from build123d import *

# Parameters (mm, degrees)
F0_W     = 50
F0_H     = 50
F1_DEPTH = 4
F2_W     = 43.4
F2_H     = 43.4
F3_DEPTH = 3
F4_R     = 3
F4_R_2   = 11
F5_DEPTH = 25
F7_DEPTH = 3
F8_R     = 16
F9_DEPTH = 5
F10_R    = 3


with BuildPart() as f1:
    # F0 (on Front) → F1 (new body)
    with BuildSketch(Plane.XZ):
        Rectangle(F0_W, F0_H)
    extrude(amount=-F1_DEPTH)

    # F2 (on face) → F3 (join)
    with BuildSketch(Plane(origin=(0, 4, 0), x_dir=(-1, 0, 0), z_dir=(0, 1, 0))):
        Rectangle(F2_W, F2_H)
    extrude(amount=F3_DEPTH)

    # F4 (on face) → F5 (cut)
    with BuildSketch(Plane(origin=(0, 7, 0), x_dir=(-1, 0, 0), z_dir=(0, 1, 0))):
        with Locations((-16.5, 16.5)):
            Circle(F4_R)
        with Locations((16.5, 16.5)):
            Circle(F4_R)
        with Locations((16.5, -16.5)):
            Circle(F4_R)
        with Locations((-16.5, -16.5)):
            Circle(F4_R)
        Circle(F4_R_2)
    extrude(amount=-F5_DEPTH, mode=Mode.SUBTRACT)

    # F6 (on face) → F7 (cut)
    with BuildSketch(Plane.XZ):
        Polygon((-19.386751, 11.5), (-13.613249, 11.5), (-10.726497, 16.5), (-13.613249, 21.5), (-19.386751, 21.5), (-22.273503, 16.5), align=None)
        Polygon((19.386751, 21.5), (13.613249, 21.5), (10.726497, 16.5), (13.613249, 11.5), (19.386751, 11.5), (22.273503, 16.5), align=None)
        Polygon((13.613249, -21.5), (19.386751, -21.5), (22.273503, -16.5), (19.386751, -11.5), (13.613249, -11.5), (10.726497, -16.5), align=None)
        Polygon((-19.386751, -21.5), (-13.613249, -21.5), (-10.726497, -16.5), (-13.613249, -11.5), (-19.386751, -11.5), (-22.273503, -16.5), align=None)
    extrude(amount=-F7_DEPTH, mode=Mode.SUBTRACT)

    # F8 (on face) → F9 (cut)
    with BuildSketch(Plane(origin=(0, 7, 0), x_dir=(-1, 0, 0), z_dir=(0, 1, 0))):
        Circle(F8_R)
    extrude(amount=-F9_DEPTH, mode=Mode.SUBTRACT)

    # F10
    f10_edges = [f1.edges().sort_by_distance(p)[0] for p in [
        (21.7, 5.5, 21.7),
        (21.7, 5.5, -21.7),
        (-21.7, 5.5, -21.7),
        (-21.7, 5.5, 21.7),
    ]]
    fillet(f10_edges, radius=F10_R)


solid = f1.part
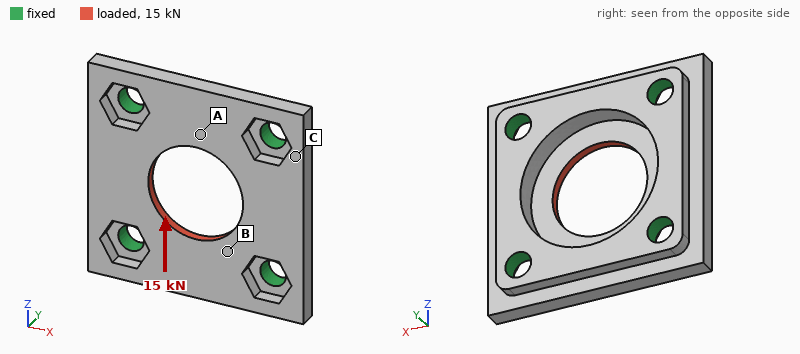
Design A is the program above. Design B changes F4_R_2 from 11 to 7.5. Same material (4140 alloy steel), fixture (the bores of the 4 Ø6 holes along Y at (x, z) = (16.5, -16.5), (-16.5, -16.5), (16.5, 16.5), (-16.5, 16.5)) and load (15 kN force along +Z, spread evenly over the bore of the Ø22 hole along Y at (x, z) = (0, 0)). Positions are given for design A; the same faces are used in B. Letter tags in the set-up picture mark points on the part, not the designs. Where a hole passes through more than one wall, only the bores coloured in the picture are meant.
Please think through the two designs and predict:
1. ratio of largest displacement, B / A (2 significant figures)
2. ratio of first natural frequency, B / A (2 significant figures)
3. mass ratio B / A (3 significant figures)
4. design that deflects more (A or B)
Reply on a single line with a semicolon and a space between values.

1.1; 0.90; 1.04; B
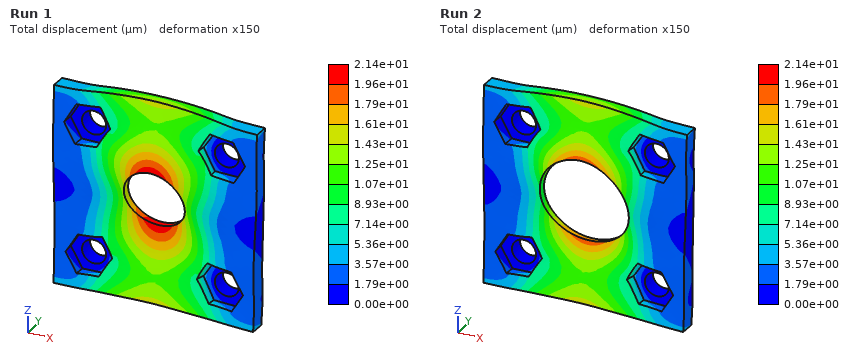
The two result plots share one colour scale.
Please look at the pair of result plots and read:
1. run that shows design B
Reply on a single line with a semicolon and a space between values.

Run 1
